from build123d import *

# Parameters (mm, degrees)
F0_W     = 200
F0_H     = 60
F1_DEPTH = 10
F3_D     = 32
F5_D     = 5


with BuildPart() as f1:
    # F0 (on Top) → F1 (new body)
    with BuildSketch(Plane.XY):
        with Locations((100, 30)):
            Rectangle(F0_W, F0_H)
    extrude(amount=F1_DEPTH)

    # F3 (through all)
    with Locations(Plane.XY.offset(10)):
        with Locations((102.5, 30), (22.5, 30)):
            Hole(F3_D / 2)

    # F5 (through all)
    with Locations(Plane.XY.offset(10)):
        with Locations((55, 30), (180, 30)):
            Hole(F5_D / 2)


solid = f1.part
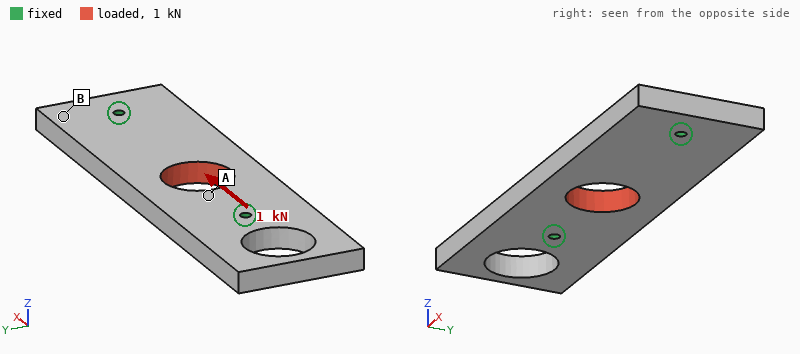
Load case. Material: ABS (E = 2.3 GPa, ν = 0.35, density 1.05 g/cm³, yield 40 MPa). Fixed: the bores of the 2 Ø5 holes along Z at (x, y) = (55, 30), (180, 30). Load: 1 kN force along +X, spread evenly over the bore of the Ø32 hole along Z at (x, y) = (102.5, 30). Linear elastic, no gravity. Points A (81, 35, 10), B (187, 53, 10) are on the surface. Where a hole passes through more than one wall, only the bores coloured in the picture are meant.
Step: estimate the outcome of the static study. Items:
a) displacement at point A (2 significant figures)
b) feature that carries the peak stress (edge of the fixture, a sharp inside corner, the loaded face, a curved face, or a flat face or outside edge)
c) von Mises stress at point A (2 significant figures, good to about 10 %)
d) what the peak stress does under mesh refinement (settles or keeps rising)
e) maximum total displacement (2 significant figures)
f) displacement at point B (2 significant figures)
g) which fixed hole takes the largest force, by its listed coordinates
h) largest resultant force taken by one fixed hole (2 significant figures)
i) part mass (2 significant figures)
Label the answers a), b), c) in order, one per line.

a) 22 µm
b) edge of the fixture
c) 1.5 MPa
d) keeps rising
e) 37 µm
f) 15 µm
g) (55, 30)
h) 550 N
i) 110 g
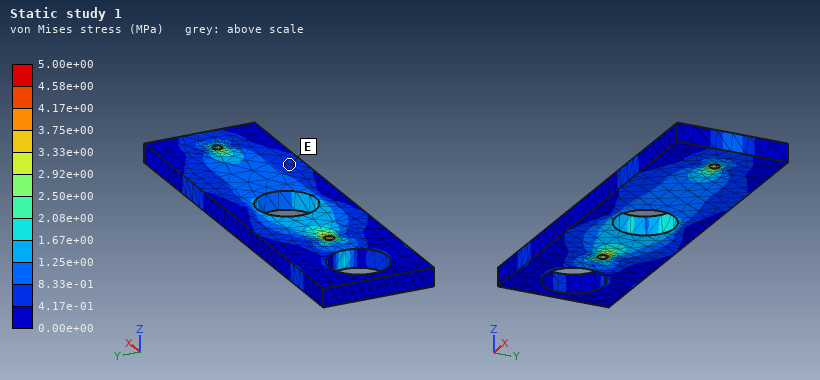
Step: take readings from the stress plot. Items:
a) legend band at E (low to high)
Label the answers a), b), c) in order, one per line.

a) 4.17e-01 to 8.33e-01 MPa
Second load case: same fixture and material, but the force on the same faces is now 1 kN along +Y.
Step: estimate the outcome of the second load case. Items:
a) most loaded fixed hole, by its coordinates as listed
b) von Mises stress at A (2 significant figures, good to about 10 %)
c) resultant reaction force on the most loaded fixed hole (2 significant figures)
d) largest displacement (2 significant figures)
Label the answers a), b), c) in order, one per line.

a) (55, 30)
b) 2.8 MPa
c) 620 N
d) 0.17 mm
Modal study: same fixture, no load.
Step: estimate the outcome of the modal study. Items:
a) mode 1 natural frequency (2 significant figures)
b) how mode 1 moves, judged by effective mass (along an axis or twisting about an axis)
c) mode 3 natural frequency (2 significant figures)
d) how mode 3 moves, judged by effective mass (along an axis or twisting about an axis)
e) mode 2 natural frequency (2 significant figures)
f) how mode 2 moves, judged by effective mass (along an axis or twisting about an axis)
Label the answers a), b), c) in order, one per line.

a) 610 Hz
b) twisting about Y
c) 900 Hz
d) twisting about X
e) 830 Hz
f) along Z
